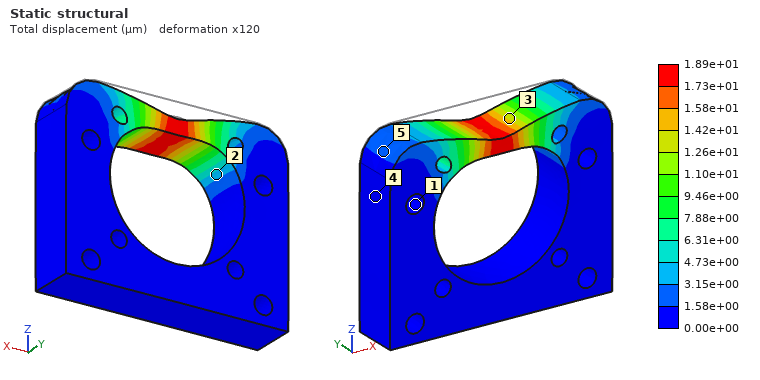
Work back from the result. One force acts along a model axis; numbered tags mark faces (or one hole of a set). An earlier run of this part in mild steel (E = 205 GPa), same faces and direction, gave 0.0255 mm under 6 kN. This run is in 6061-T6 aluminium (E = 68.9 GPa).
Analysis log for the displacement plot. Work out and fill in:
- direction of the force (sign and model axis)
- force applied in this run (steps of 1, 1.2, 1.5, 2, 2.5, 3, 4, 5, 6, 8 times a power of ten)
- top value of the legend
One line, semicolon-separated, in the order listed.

-Z; 1.5 kN; 1.89e+01 µm
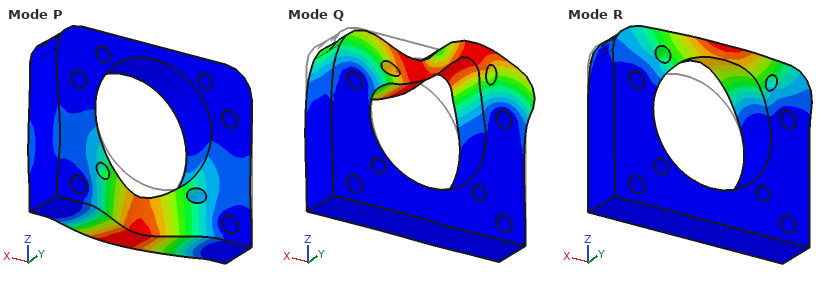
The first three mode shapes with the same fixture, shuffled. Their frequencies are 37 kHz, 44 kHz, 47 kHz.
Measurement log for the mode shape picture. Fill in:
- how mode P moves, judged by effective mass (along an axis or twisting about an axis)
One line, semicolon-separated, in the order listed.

along Y
